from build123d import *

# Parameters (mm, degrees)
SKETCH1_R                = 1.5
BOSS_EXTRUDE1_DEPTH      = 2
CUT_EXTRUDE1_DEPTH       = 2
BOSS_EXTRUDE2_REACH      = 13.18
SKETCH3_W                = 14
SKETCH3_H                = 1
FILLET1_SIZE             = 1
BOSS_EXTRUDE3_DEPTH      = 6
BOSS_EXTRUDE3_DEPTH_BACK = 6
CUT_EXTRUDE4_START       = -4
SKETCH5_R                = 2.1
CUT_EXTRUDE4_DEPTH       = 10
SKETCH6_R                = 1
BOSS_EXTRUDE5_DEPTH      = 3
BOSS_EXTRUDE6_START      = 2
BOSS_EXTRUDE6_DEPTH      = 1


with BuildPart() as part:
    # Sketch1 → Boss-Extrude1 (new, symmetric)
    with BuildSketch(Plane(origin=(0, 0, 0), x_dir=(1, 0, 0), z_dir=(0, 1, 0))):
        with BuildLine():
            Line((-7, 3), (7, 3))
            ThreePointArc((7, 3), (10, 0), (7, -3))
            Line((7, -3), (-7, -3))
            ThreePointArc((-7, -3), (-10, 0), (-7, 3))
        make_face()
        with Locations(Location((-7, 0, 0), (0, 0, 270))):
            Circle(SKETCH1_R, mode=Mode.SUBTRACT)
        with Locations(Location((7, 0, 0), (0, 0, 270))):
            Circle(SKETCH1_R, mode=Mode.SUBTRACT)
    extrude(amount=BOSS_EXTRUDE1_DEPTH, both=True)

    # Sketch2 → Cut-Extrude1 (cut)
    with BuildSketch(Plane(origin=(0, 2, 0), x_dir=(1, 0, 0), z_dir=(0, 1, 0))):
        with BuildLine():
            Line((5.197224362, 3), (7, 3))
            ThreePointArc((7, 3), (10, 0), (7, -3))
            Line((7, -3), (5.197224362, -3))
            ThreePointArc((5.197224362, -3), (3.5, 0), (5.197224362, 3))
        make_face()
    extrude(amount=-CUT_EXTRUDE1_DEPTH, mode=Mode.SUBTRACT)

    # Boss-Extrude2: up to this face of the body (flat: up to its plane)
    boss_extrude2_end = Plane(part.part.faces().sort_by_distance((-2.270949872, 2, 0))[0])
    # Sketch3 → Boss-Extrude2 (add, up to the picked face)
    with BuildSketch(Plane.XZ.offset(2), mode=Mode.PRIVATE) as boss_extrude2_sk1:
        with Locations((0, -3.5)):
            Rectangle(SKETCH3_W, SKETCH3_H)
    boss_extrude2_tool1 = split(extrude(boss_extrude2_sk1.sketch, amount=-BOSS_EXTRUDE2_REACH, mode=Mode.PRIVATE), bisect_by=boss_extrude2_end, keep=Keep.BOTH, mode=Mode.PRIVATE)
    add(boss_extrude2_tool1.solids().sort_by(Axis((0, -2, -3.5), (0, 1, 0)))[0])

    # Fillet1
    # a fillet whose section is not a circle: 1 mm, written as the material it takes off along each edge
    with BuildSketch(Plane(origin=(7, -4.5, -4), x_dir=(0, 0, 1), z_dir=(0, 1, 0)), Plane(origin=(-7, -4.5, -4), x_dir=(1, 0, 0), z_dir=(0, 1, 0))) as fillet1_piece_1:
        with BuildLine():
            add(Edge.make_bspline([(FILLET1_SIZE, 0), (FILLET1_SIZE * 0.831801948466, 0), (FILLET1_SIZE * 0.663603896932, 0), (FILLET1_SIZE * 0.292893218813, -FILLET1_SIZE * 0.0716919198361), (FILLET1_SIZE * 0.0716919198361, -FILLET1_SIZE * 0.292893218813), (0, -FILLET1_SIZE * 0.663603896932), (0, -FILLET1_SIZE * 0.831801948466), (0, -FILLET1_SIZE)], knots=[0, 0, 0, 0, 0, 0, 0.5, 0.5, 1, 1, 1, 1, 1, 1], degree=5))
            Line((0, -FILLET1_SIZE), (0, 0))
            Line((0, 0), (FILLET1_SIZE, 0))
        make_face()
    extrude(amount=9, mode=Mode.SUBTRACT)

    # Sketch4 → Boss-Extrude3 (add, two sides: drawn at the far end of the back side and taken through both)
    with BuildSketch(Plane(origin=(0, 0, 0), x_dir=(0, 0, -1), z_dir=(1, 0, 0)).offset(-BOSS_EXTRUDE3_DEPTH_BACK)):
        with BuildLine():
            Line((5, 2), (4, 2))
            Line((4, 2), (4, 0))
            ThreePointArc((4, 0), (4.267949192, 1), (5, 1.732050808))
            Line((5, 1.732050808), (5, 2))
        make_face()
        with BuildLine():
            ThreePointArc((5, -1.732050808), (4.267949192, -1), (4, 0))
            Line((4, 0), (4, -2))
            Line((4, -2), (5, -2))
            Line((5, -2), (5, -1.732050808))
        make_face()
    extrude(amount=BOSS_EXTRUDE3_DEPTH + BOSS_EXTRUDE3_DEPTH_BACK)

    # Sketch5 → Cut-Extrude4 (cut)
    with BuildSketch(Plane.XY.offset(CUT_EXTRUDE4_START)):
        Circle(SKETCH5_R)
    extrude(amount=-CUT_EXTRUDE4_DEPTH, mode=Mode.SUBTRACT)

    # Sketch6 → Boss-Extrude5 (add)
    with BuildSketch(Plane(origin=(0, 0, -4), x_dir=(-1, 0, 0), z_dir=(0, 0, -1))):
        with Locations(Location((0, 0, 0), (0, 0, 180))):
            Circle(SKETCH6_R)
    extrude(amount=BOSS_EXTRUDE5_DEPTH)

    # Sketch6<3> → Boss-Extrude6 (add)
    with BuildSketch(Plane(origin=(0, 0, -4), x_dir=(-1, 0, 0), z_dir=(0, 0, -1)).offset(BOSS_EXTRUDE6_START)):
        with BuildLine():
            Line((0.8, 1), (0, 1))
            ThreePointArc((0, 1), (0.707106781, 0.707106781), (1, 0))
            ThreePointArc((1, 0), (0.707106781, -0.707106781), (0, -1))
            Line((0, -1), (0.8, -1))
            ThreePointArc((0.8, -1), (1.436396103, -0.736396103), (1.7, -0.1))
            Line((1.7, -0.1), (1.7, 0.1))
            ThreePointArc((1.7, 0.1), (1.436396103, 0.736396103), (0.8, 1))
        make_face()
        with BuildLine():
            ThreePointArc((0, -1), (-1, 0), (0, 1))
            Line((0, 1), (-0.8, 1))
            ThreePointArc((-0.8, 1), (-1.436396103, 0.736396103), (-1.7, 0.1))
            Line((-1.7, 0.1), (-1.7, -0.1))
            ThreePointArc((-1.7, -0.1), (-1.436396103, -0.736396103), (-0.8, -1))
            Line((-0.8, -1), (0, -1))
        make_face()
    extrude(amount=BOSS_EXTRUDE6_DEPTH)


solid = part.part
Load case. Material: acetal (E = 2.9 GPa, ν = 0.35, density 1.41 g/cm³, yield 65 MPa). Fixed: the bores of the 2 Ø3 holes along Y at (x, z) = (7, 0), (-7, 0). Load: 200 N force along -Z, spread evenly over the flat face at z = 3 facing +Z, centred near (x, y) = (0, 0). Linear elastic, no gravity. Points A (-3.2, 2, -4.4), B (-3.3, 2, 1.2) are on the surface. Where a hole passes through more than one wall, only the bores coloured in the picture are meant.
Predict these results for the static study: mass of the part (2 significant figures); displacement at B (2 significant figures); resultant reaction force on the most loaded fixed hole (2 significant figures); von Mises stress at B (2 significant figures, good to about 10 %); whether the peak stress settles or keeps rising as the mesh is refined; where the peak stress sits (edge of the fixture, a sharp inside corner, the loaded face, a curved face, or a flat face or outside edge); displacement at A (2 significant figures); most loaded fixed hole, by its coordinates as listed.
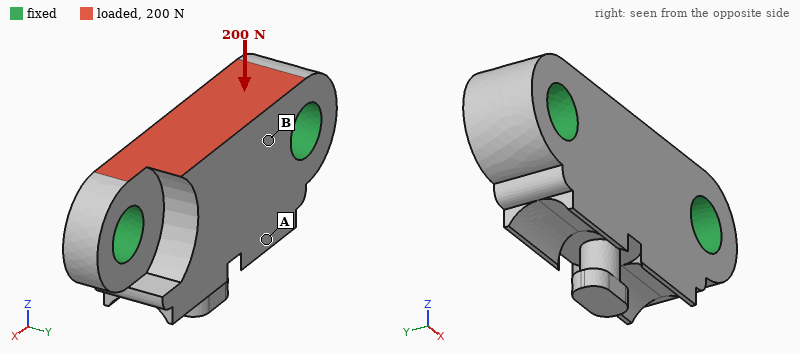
0.60 g
17 µm
110 N
7.1 MPa
keeps rising
edge of the fixture
18 µm
(-7, 0)
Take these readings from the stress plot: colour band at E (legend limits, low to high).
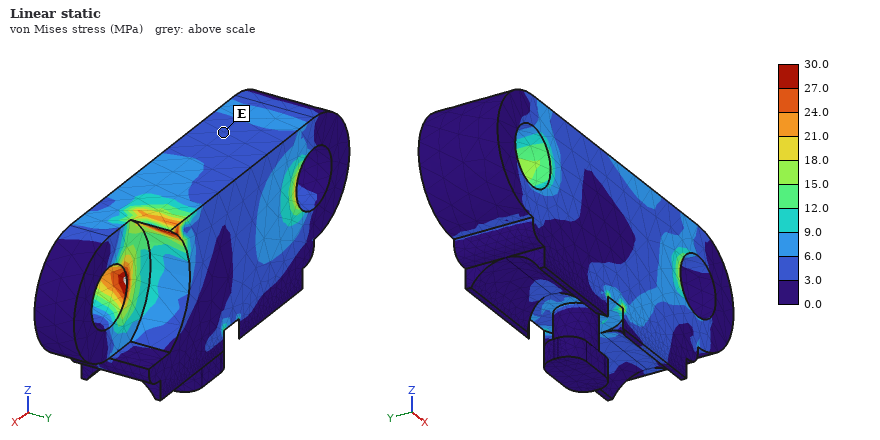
3.0 to 6.0 MPa
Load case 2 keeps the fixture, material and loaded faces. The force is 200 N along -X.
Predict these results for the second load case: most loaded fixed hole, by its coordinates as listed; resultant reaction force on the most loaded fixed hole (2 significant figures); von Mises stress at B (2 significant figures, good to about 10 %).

(-7, 0)
130 N
5.2 MPa
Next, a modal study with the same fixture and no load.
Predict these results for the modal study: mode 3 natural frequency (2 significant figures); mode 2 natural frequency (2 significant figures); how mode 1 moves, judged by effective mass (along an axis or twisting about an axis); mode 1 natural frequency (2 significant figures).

22 kHz
21 kHz
along Y
15 kHz
